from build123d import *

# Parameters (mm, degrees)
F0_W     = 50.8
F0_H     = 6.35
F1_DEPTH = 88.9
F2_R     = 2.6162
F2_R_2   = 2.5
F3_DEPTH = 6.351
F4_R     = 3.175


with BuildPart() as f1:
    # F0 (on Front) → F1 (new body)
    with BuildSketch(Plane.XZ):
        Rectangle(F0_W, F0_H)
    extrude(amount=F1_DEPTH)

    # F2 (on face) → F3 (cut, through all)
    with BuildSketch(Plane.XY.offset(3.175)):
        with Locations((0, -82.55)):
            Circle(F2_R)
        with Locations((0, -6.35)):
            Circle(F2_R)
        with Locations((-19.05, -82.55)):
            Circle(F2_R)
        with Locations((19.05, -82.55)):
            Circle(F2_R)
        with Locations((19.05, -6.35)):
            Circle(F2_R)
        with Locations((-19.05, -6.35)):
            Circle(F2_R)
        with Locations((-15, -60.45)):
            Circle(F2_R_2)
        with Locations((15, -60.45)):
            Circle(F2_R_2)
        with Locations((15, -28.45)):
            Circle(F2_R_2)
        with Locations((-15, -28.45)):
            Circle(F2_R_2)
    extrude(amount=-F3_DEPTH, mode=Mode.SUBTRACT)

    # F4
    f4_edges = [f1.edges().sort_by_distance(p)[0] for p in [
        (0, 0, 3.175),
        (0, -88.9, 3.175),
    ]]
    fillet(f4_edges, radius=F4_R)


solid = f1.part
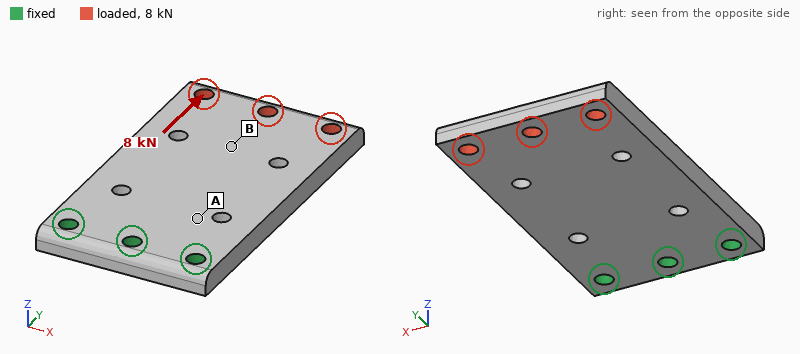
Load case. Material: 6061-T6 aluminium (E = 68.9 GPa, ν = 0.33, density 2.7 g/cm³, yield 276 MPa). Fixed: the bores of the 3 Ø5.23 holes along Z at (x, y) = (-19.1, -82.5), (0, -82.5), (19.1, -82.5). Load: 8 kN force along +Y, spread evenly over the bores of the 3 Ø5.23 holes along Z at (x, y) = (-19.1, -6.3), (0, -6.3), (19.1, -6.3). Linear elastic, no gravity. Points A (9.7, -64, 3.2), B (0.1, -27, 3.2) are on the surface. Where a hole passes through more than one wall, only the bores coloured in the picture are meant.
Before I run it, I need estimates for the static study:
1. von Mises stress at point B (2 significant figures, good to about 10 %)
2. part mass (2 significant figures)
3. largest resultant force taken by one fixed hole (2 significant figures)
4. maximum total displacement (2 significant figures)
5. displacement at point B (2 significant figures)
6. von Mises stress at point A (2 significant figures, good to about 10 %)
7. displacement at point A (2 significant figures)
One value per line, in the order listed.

24 MPa
73 g
2.8 kN
35 µm
21 µm
30 MPa
7.2 µm
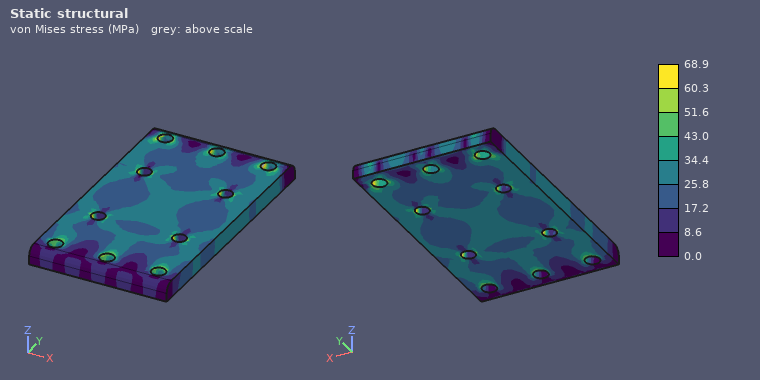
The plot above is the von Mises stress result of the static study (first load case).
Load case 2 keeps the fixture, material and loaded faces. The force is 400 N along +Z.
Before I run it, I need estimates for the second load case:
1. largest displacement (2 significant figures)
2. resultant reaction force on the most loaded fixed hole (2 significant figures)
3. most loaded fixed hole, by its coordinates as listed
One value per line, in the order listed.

0.88 mm
370 N
(0, -82.5)
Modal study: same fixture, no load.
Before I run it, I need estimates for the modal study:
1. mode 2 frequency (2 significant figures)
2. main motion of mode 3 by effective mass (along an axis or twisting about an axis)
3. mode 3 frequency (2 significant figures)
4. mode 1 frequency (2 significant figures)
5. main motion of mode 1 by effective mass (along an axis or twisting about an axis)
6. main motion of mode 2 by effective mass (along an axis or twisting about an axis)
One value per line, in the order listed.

2700 Hz
along Z
4800 Hz
800 Hz
along Z
twisting about Y
